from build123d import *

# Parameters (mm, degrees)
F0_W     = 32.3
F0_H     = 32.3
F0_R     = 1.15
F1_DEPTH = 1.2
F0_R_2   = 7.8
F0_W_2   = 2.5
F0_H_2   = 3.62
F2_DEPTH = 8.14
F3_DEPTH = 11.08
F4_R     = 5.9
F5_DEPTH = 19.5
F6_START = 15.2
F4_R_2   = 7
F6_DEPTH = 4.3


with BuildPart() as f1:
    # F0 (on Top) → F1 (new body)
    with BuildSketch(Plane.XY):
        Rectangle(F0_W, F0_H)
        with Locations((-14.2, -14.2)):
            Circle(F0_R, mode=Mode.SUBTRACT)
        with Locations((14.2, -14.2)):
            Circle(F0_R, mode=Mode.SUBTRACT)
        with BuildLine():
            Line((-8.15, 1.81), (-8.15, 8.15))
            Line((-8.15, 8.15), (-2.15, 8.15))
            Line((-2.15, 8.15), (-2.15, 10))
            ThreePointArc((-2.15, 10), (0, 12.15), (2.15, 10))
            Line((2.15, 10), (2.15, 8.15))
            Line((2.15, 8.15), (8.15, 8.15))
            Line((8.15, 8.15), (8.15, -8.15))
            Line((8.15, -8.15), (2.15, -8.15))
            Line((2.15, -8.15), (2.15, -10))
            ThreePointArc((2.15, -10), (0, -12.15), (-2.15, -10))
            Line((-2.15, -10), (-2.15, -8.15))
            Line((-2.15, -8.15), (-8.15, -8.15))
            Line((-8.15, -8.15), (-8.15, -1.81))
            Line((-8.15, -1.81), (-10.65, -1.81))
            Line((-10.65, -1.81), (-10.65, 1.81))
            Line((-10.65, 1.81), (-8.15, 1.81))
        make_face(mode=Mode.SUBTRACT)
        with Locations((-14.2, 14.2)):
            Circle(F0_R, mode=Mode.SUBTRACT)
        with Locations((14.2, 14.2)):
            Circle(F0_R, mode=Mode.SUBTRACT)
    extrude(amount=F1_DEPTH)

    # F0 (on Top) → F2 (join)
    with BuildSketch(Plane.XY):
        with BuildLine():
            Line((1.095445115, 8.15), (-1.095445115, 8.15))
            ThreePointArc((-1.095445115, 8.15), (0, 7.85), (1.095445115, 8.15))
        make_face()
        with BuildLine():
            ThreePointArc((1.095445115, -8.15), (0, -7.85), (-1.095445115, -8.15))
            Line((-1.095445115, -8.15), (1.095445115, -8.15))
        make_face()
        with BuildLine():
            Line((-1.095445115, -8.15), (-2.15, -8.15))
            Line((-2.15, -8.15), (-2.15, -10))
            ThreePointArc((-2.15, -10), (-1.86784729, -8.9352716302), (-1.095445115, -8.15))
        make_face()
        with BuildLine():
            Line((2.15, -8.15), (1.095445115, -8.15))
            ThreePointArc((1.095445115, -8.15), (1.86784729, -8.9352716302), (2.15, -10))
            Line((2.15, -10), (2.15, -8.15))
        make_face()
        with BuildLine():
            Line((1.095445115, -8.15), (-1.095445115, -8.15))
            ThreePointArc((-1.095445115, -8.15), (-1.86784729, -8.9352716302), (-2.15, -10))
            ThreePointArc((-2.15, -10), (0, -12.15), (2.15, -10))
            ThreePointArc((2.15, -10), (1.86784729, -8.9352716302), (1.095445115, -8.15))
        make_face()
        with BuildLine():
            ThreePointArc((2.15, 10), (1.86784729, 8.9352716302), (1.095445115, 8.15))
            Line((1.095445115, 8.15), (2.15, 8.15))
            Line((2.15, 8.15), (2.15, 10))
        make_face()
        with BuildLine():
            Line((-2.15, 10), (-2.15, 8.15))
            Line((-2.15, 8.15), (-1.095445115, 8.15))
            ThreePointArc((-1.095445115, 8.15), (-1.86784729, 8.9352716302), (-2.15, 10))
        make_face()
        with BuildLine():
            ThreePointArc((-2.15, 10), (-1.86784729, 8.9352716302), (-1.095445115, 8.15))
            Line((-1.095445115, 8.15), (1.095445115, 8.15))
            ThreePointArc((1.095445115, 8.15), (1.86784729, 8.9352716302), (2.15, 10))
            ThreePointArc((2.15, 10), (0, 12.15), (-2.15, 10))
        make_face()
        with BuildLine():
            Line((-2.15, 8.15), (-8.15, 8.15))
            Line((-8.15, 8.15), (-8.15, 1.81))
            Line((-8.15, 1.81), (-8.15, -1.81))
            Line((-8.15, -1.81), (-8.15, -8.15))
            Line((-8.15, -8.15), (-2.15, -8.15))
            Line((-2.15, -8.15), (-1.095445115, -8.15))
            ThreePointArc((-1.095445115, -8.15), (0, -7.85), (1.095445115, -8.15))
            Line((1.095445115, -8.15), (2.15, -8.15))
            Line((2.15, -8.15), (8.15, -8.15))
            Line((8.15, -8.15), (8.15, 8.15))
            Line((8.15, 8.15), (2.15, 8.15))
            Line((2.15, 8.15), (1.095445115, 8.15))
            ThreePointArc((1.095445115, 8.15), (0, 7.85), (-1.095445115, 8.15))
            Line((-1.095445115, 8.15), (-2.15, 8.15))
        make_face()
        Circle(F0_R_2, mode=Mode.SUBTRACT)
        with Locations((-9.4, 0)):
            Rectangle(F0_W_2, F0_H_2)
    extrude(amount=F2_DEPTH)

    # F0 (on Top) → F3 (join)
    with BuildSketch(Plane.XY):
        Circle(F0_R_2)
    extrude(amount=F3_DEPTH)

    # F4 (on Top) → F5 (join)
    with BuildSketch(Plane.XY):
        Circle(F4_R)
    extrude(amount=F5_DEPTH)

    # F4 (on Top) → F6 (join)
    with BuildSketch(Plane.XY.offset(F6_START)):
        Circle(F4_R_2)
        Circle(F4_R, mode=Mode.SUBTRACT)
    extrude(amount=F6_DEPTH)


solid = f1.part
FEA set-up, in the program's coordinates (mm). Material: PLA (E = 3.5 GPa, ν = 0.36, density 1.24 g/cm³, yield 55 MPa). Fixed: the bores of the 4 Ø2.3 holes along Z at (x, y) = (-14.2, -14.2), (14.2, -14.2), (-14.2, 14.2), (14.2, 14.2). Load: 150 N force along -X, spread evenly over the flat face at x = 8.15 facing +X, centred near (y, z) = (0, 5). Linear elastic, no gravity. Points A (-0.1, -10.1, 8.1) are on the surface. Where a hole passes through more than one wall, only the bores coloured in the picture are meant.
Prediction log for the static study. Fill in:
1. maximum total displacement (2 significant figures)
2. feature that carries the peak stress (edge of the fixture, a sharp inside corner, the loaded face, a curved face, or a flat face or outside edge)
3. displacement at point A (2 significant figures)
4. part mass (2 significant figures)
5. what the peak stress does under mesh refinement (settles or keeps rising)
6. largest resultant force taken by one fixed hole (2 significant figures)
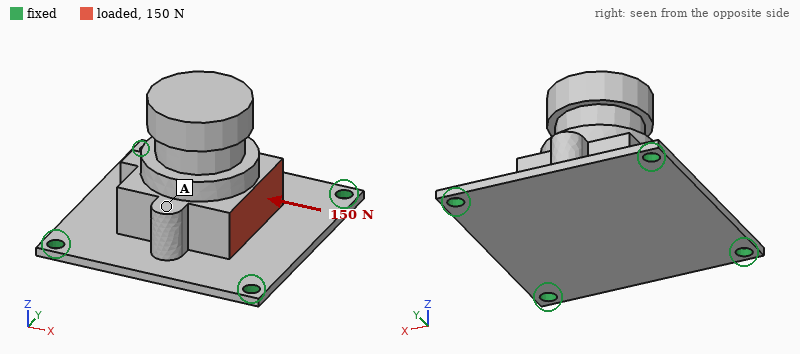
0.34 mm
edge of the fixture
0.14 mm
6.2 g
keeps rising
44 N
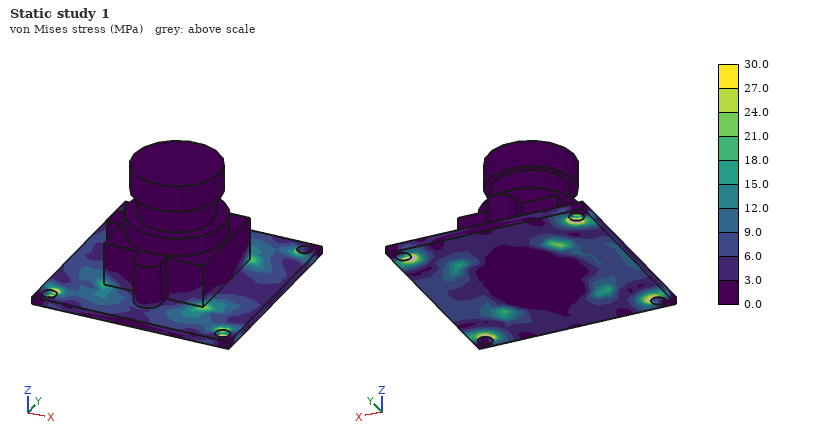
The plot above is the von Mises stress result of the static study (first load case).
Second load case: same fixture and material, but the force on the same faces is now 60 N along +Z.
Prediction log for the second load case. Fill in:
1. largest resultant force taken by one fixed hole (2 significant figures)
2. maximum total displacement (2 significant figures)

26 N
0.39 mm
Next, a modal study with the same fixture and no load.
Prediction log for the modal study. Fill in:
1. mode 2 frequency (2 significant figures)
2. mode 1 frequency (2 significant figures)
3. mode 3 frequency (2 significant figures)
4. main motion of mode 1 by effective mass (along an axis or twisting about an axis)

1300 Hz
1100 Hz
1300 Hz
along Z
